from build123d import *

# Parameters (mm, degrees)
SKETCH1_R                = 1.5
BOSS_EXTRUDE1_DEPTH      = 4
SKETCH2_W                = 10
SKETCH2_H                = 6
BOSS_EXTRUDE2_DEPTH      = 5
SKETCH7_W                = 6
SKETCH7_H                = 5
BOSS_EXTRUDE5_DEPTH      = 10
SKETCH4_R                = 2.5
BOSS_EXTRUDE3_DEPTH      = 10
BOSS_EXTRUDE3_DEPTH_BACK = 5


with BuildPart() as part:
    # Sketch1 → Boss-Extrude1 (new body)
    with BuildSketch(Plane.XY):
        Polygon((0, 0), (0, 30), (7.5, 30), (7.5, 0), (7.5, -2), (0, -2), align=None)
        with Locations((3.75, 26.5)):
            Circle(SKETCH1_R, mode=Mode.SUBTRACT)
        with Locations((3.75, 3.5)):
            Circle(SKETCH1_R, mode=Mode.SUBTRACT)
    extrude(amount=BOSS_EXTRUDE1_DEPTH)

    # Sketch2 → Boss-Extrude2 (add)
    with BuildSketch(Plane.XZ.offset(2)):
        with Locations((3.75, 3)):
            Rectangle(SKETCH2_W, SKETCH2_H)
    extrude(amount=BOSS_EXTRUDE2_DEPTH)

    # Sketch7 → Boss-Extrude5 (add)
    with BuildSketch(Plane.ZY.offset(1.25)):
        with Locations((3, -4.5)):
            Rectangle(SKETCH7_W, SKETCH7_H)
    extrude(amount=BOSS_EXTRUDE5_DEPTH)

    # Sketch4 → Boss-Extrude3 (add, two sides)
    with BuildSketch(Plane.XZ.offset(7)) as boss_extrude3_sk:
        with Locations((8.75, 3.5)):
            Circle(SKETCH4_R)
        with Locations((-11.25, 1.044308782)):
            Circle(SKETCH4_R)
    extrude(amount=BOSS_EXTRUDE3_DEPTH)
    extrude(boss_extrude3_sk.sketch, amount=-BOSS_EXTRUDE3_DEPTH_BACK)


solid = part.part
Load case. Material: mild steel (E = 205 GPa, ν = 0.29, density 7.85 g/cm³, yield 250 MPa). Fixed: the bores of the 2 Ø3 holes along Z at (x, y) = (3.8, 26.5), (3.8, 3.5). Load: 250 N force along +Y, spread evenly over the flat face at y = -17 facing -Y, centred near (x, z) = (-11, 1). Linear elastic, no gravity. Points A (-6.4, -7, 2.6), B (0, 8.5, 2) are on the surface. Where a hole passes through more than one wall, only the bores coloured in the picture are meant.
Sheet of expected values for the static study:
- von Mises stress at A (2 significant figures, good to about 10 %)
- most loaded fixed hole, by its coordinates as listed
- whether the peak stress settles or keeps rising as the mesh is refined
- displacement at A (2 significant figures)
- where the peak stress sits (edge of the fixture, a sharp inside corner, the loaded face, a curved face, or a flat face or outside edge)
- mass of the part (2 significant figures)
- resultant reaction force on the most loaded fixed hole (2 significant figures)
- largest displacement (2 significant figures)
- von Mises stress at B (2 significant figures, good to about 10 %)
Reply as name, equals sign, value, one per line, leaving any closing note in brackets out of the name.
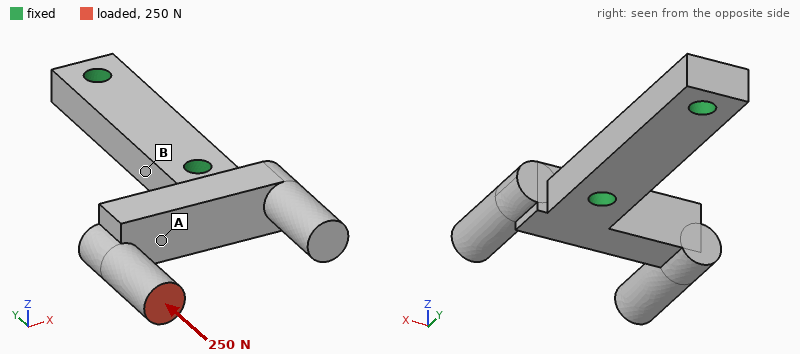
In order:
von Mises stress at A = 58 MPa
most loaded fixed hole, by its coordinates as listed = (3.8, 3.5)
whether the peak stress settles or keeps rising as the mesh is refined = keeps rising
displacement at A = 23 µm
where the peak stress sits = a sharp inside corner
mass of the part = 16 g
resultant reaction force on the most loaded fixed hole = 250 N
largest displacement = 62 µm
von Mises stress at B = 16 MPa
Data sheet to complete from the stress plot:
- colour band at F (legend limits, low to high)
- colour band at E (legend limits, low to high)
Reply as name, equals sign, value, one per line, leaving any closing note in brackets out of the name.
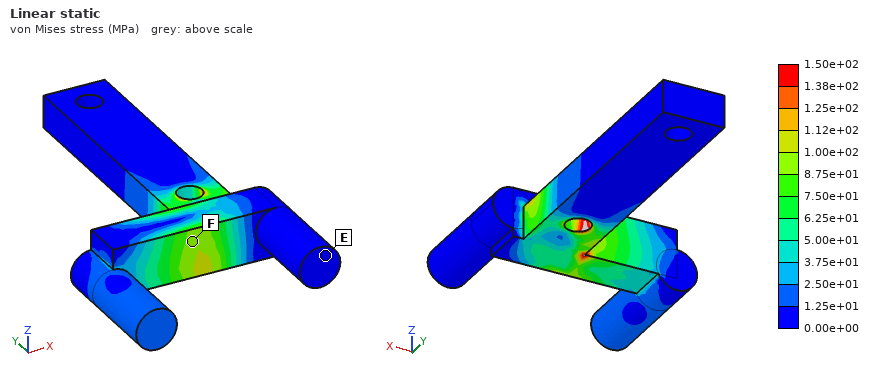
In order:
colour band at F = 8.75e+01 to 1.00e+02 MPa
colour band at E = 0.00e+00 to 1.25e+01 MPa
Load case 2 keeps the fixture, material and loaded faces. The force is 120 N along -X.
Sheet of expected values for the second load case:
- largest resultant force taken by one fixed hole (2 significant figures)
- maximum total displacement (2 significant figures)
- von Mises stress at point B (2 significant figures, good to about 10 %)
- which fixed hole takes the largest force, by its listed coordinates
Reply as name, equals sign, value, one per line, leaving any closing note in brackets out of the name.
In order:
largest resultant force taken by one fixed hole = 150 N
maximum total displacement = 53 µm
von Mises stress at point B = 10 MPa
which fixed hole takes the largest force, by its listed coordinates = (3.8, 3.5)
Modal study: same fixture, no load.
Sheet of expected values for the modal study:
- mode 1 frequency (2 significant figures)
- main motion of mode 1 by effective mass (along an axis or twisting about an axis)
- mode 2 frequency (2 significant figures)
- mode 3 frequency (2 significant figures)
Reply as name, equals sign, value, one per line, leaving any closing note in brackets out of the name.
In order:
mode 1 frequency = 5100 Hz
main motion of mode 1 by effective mass = along Z
mode 2 frequency = 6000 Hz
mode 3 frequency = 8700 Hz
